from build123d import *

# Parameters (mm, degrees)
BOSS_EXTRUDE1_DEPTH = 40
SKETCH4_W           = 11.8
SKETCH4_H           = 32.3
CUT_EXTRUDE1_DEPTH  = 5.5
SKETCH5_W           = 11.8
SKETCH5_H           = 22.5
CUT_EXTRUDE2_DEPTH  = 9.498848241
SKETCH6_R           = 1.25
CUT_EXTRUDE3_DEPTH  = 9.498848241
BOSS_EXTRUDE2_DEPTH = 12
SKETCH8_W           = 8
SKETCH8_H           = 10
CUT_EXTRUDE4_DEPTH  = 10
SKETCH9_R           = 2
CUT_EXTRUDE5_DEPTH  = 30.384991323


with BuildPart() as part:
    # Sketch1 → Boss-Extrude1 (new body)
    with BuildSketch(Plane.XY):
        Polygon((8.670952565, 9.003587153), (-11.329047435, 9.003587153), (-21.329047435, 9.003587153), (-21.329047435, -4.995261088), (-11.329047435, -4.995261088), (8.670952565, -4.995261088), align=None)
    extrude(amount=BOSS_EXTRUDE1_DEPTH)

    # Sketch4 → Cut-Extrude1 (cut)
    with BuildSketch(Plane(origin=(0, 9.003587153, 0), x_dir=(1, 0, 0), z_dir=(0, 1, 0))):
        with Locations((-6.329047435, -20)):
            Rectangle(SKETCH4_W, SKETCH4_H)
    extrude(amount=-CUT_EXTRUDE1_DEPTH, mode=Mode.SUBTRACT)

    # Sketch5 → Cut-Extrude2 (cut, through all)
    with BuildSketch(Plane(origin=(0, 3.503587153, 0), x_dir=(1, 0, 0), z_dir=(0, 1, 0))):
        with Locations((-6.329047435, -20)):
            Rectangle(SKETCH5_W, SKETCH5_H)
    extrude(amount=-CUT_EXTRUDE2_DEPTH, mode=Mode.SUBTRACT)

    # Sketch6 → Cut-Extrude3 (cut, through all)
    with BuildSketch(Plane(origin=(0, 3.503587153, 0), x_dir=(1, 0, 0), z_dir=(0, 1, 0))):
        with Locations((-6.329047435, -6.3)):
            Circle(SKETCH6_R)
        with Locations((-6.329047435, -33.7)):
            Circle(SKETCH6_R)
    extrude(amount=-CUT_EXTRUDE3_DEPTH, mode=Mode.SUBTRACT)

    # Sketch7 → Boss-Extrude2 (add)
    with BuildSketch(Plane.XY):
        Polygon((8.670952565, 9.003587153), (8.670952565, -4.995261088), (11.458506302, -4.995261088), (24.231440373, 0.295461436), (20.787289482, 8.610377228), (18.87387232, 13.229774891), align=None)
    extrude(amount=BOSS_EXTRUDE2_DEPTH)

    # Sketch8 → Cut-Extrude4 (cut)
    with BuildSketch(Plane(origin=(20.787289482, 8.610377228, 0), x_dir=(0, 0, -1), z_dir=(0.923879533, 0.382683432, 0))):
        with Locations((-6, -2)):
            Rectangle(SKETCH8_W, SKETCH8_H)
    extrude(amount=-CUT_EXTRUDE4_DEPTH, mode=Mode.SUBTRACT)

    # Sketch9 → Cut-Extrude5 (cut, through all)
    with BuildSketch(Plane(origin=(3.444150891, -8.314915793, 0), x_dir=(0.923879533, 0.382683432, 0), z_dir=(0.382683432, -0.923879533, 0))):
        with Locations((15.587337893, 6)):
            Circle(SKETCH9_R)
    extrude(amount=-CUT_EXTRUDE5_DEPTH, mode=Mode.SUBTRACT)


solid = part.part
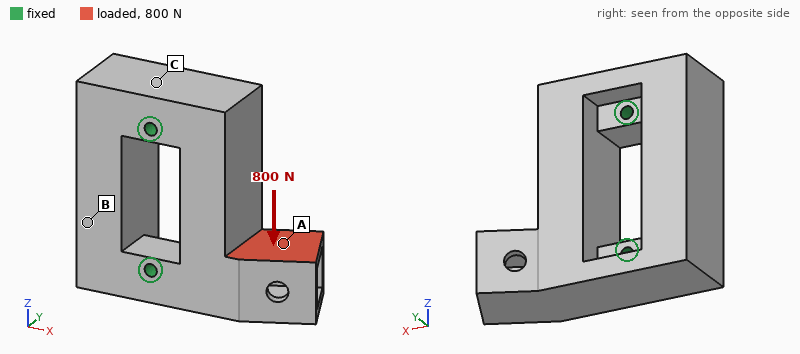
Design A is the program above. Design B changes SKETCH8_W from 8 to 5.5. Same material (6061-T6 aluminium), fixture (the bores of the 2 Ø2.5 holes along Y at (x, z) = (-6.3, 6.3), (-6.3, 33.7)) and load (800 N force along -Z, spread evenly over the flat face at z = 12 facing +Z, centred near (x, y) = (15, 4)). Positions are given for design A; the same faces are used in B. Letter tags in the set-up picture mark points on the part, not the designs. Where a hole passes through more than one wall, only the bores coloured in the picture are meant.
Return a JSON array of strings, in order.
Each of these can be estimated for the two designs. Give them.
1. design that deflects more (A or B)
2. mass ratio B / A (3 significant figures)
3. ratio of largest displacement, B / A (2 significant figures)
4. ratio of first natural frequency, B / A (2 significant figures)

["A", "1.02", "0.81", "0.95"]
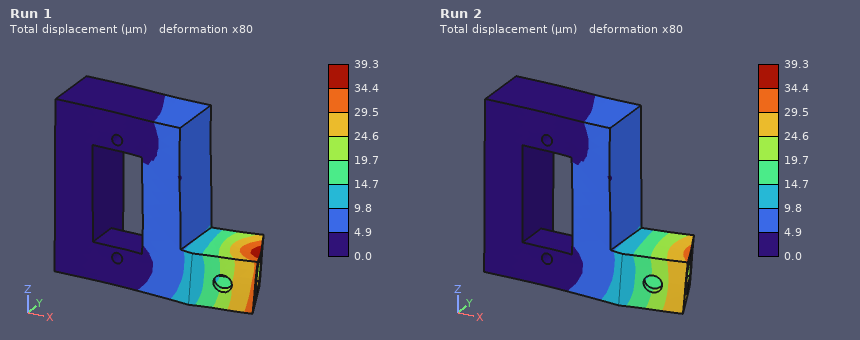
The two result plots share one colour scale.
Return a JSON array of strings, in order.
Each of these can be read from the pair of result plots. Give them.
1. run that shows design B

["Run 2"]
